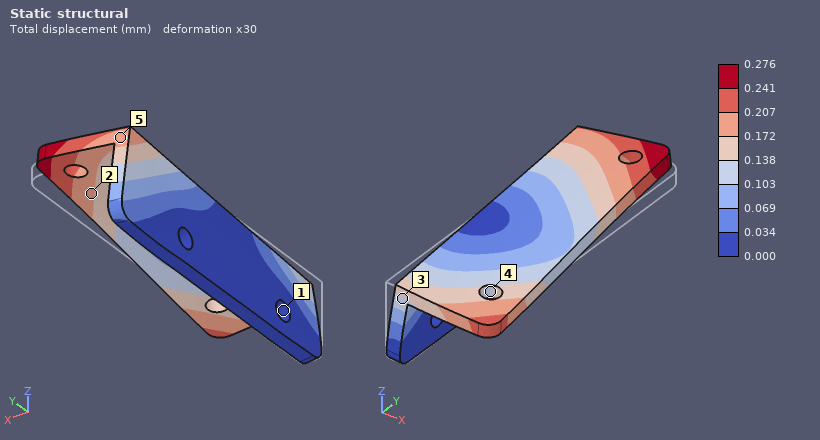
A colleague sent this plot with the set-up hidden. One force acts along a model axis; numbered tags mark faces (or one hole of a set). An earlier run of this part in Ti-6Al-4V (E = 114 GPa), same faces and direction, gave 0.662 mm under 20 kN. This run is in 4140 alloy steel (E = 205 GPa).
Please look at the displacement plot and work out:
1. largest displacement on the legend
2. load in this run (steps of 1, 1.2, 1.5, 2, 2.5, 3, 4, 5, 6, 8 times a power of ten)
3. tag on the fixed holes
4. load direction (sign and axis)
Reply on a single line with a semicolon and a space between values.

0.276 mm; 15 kN; 1; +Y
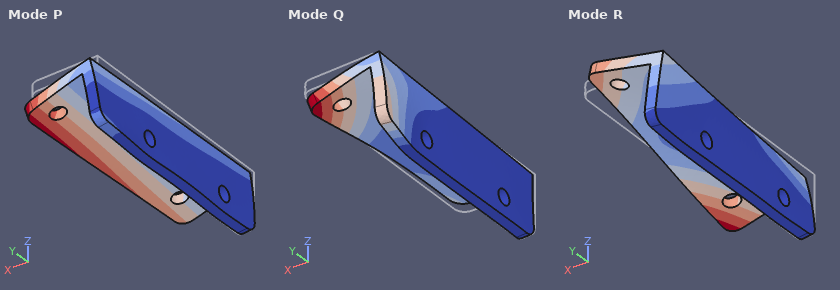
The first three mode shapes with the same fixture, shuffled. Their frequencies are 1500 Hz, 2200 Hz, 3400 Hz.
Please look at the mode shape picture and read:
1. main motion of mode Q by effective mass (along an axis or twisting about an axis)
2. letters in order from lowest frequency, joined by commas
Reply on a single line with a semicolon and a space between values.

along X; P, R, Q
